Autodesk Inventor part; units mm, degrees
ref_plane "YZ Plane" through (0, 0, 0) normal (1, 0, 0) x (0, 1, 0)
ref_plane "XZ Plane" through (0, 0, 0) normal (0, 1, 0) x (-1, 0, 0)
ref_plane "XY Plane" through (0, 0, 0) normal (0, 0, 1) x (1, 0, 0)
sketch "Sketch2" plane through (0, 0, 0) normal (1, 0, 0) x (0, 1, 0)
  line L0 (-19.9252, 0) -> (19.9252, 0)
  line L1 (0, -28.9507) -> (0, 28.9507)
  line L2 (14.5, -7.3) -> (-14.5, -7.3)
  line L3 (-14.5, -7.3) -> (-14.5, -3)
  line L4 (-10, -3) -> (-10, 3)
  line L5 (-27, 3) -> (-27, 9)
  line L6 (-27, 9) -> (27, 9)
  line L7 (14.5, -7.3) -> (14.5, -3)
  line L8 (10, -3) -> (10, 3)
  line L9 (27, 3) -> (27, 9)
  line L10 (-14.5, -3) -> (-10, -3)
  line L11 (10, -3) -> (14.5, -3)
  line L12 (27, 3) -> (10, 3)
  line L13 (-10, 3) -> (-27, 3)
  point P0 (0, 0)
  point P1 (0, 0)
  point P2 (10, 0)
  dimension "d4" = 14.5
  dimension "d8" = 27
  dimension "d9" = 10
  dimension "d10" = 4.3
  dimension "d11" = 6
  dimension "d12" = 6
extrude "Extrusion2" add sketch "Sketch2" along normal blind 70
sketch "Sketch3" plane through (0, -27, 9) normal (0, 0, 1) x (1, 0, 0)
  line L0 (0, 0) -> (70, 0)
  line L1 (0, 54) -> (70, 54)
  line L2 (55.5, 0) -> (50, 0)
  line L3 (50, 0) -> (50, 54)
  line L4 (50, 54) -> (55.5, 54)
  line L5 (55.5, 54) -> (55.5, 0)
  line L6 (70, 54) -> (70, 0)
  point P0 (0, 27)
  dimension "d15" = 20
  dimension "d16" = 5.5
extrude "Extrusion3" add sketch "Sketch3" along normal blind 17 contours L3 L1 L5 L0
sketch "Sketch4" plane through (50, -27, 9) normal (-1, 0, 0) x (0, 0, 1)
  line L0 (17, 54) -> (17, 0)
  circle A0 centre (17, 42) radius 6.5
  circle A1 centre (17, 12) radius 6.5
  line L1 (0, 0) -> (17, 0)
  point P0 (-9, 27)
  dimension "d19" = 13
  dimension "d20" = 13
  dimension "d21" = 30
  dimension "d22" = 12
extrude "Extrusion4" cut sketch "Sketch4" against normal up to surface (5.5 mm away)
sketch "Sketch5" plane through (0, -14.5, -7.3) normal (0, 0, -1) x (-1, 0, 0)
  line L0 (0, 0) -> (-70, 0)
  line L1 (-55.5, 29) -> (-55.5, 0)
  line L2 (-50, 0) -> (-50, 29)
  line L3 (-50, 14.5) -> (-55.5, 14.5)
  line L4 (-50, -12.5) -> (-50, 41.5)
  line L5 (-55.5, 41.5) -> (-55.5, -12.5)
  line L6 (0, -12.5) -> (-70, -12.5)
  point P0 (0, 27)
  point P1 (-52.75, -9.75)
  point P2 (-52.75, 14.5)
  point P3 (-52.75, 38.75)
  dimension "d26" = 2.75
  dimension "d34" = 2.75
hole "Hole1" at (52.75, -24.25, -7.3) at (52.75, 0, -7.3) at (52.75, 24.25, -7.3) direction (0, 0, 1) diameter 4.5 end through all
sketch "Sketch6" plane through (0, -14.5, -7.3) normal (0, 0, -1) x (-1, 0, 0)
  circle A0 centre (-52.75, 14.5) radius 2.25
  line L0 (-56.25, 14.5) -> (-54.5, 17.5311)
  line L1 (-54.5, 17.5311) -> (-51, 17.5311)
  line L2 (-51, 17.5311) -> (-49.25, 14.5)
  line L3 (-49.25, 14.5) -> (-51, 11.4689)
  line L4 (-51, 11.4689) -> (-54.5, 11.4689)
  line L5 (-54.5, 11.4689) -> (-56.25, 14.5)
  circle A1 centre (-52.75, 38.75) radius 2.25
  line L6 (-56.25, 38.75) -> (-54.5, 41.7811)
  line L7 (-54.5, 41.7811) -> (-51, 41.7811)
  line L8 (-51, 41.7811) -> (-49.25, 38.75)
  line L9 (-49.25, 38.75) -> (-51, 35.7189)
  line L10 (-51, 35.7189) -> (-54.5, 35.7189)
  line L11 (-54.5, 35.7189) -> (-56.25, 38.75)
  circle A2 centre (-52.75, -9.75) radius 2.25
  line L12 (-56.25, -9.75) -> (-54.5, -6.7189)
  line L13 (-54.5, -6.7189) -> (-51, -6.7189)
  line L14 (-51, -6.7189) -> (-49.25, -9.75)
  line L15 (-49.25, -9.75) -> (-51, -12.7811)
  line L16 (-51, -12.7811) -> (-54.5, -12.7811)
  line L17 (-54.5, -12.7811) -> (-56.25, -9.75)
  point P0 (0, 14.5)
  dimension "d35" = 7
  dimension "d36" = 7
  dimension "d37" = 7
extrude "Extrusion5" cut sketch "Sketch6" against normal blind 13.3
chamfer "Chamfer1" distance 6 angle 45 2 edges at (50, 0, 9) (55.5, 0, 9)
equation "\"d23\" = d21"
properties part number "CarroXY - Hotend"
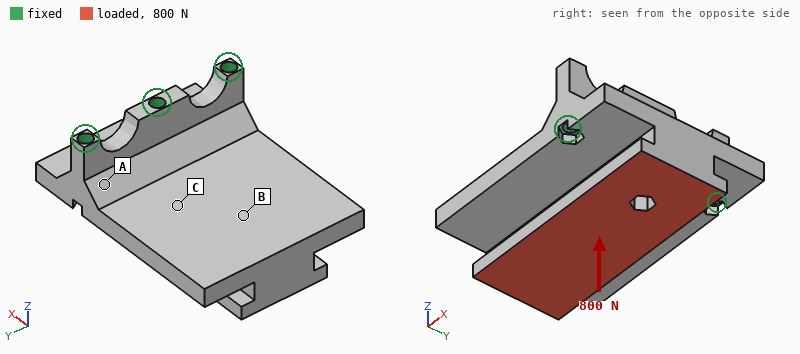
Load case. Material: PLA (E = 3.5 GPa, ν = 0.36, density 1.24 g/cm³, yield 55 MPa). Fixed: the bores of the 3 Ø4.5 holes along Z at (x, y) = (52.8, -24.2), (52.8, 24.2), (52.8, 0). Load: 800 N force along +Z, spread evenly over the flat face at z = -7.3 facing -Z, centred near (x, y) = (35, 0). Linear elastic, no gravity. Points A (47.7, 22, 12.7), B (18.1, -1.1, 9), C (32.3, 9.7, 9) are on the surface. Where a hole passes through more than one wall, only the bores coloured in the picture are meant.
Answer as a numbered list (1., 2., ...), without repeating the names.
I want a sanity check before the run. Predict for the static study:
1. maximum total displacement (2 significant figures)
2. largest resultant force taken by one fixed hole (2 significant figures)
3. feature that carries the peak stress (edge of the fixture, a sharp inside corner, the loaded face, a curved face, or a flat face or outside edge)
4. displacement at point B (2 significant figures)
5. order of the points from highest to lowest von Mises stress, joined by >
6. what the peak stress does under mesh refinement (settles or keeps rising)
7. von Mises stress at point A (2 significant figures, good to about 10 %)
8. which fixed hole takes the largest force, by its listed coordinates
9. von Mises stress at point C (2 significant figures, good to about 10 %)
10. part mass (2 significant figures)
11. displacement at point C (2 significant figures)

1. 0.69 mm
2. 580 N
3. edge of the fixture
4. 0.41 mm
5. A > C > B
6. keeps rising
7. 12 MPa
8. (52.8, 0)
9. 5.0 MPa
10. 55 g
11. 0.21 mm
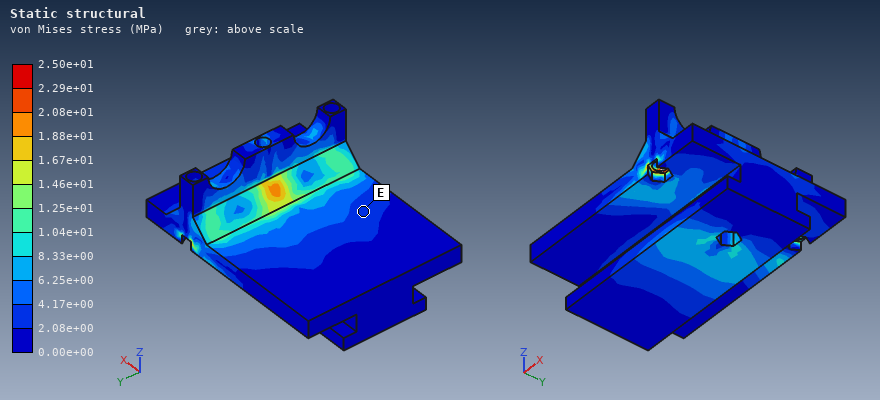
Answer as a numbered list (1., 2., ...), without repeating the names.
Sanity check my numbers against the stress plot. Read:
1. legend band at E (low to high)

1. 2.08e+00 to 4.17e+00 MPa
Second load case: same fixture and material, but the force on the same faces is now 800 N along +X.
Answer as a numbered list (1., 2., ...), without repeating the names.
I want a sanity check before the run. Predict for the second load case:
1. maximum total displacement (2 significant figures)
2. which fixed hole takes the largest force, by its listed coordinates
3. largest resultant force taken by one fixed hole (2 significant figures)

1. 0.55 mm
2. (52.8, 0)
3. 500 N
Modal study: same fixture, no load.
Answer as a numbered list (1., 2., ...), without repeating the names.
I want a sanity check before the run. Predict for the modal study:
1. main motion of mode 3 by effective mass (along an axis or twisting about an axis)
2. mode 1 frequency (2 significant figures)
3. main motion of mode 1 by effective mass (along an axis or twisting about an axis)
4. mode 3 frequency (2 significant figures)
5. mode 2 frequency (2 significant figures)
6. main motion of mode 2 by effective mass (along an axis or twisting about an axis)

1. along Y
2. 920 Hz
3. along Z
4. 2700 Hz
5. 2200 Hz
6. twisting about X
